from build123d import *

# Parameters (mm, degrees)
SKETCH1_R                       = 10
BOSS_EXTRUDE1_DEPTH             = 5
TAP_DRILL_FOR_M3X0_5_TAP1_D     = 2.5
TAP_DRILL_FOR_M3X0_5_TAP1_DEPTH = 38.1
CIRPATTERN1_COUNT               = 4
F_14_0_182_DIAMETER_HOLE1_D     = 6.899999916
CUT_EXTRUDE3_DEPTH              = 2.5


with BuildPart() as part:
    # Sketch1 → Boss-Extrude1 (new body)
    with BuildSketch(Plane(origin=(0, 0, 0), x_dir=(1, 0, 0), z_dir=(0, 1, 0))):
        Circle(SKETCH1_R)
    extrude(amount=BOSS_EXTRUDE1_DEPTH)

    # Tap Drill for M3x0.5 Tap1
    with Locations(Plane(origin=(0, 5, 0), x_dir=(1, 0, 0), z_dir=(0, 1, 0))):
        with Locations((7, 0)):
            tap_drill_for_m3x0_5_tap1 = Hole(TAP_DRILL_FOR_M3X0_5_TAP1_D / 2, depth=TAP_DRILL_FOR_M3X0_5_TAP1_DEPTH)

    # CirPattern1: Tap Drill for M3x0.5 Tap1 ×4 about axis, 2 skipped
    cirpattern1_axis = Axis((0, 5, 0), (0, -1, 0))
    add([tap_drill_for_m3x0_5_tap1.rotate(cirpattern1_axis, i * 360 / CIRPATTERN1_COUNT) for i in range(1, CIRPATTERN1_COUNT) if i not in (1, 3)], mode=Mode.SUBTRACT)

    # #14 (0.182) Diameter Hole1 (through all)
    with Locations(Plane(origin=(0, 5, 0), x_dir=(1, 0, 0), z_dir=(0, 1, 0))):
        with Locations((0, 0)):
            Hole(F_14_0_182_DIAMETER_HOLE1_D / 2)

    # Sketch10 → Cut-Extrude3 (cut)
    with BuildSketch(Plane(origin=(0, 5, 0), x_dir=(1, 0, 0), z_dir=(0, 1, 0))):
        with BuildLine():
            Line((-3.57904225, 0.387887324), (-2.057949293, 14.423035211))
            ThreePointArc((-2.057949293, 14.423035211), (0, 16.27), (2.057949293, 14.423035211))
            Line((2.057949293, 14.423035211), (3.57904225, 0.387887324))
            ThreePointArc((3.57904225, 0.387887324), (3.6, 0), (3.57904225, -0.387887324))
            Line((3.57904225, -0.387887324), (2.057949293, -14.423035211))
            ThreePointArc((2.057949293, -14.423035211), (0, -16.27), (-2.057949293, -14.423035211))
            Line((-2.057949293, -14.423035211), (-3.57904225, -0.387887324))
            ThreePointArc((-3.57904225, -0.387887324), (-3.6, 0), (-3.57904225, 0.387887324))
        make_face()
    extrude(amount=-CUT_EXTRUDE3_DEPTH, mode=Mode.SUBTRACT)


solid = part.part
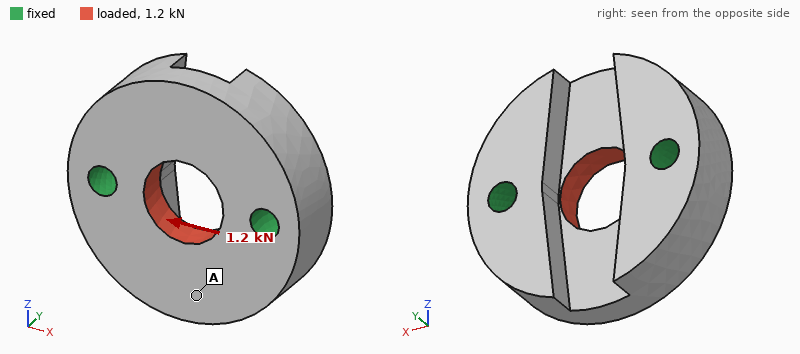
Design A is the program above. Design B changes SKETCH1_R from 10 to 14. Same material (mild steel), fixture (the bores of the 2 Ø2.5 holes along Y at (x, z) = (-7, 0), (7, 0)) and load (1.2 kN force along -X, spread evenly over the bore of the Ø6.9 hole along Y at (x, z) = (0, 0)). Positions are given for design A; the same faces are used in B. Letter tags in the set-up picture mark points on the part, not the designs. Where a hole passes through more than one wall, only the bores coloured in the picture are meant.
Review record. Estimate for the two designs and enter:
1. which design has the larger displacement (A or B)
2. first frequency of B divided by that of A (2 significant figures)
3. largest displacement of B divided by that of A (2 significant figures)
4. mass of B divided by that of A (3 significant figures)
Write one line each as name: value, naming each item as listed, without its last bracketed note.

which design has the larger displacement: A
first frequency of B divided by that of A: 0.53
largest displacement of B divided by that of A: 0.85
mass of B divided by that of A: 2.26
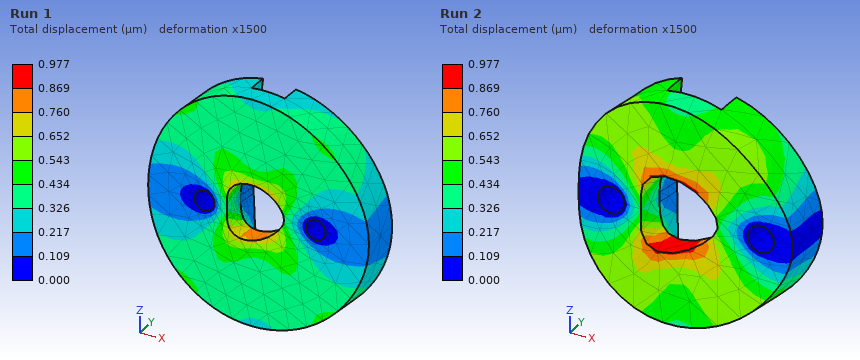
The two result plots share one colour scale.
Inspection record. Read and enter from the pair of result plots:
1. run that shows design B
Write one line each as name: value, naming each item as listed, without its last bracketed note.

run that shows design B: Run 1
